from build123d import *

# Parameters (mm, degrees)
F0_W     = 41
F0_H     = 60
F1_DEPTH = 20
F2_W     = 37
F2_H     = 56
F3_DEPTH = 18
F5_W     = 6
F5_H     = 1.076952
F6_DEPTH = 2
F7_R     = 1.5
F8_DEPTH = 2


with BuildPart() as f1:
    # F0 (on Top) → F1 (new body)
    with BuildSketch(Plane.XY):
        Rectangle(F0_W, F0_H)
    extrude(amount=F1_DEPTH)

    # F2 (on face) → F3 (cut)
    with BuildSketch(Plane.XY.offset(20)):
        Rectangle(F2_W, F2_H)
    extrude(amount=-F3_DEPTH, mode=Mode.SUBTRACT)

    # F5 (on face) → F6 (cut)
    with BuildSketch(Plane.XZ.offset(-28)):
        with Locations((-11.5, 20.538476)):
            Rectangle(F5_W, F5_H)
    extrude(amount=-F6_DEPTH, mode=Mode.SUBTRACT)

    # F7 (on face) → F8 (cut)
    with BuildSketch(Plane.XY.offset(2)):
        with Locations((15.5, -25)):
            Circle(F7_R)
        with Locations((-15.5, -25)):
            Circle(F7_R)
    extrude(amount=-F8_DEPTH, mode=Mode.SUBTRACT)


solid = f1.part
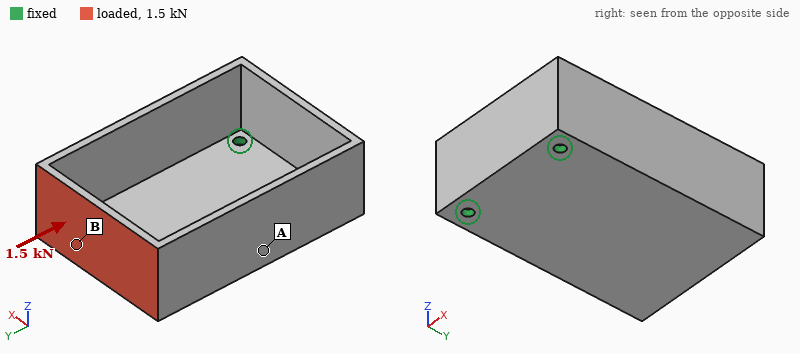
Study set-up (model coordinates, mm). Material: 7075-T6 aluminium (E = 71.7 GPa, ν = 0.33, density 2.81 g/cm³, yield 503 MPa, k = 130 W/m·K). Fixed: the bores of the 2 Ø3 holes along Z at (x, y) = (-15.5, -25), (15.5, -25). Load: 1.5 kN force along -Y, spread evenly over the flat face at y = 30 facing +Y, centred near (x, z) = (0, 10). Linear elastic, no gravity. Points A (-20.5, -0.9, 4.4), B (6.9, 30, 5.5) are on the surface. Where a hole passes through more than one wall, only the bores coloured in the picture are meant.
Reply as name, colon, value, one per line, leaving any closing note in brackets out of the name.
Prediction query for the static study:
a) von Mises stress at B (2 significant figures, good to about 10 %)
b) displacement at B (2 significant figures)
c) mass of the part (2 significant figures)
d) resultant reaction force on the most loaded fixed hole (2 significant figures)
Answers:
von Mises stress at B: 76 MPa
displacement at B: 0.72 mm
mass of the part: 33 g
resultant reaction force on the most loaded fixed hole: 750 N
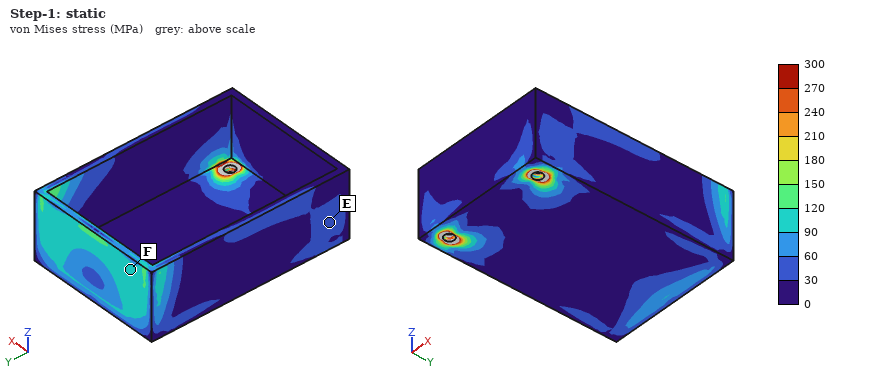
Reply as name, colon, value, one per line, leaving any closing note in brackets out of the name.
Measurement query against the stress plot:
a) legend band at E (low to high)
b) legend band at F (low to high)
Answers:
legend band at E: 30 to 60 MPa
legend band at F: 90 to 120 MPa
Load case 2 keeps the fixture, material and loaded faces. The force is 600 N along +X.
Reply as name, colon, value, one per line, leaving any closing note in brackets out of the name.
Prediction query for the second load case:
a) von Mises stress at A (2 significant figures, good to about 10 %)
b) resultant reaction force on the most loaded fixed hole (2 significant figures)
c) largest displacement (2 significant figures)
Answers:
von Mises stress at A: 43 MPa
resultant reaction force on the most loaded fixed hole: 1.1 kN
largest displacement: 0.57 mm
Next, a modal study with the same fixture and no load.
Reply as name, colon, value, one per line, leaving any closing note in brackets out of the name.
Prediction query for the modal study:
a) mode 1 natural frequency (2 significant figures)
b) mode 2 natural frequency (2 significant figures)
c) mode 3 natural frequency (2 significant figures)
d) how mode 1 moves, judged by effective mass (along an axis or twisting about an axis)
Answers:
mode 1 natural frequency: 840 Hz
mode 2 natural frequency: 1400 Hz
mode 3 natural frequency: 4500 Hz
how mode 1 moves, judged by effective mass: along Z
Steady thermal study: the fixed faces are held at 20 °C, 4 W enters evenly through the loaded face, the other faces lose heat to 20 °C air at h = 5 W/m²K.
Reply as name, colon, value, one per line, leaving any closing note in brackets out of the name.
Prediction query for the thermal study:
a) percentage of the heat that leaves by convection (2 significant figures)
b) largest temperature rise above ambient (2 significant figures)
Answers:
percentage of the heat that leaves by convection: 8.6 %
largest temperature rise above ambient: 14 K
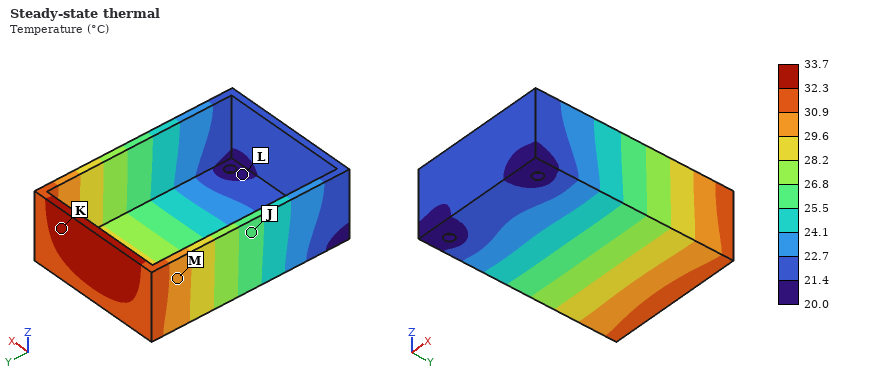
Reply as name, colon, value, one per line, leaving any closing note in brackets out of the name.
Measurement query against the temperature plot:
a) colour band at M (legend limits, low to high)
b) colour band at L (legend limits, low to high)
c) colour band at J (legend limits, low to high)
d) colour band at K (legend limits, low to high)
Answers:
colour band at M: 29.6 to 30.9 °C
colour band at L: 20.0 to 21.4 °C
colour band at J: 25.5 to 26.8 °C
colour band at K: 32.3 to 33.7 °C
